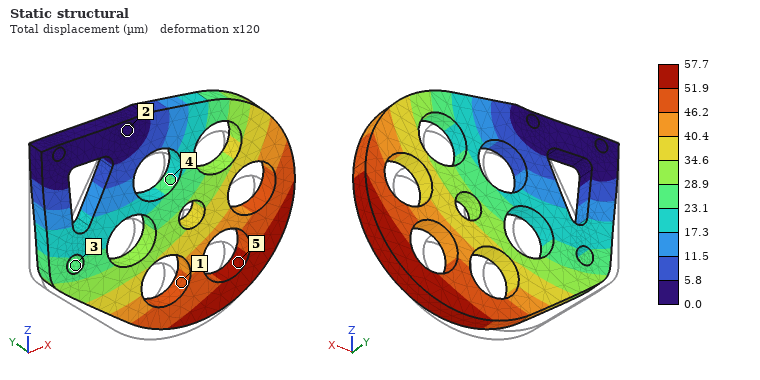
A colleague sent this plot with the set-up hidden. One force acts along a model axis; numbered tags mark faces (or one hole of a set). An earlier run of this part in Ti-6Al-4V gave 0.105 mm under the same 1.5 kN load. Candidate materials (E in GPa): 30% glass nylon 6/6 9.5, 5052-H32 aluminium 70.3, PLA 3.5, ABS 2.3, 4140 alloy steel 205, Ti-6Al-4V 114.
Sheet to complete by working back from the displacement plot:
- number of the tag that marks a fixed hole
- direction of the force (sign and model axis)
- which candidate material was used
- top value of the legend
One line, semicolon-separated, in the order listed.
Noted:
2; +X; 4140 alloy steel; 57.7 µm
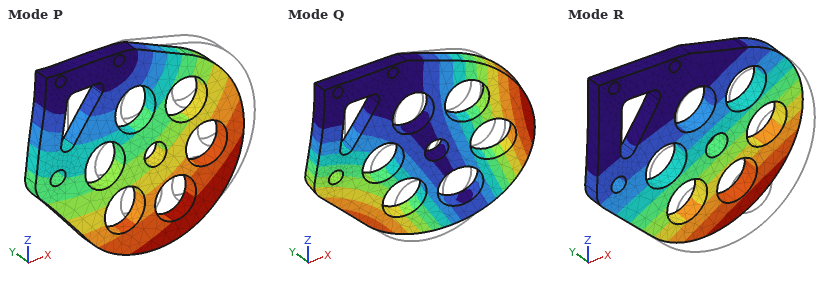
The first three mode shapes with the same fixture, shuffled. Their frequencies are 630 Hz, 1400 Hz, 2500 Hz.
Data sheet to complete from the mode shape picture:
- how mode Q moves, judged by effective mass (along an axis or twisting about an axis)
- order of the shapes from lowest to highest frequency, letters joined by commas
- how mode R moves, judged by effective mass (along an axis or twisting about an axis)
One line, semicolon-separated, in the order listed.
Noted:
twisting about Z; R, Q, P; along Y
